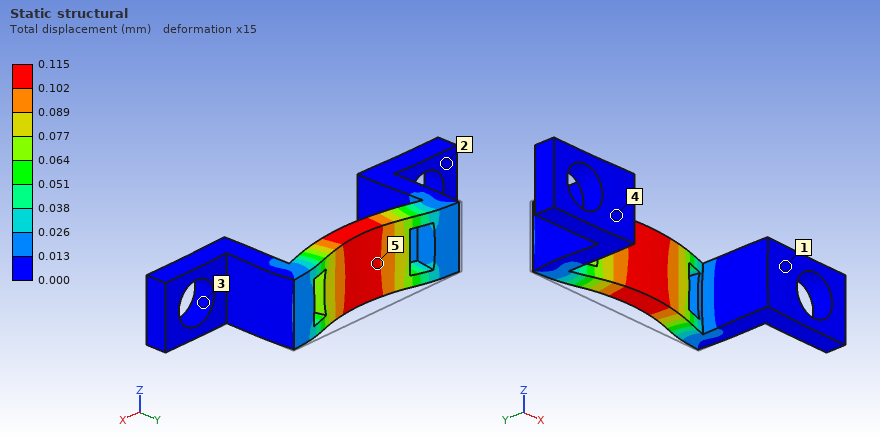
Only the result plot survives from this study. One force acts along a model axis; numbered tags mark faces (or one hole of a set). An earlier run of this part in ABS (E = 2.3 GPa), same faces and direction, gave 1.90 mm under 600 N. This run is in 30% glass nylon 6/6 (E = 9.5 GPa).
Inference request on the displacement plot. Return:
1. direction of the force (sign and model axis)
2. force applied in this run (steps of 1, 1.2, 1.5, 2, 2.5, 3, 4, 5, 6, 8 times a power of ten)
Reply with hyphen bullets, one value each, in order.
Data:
- -Y
- 150 N
